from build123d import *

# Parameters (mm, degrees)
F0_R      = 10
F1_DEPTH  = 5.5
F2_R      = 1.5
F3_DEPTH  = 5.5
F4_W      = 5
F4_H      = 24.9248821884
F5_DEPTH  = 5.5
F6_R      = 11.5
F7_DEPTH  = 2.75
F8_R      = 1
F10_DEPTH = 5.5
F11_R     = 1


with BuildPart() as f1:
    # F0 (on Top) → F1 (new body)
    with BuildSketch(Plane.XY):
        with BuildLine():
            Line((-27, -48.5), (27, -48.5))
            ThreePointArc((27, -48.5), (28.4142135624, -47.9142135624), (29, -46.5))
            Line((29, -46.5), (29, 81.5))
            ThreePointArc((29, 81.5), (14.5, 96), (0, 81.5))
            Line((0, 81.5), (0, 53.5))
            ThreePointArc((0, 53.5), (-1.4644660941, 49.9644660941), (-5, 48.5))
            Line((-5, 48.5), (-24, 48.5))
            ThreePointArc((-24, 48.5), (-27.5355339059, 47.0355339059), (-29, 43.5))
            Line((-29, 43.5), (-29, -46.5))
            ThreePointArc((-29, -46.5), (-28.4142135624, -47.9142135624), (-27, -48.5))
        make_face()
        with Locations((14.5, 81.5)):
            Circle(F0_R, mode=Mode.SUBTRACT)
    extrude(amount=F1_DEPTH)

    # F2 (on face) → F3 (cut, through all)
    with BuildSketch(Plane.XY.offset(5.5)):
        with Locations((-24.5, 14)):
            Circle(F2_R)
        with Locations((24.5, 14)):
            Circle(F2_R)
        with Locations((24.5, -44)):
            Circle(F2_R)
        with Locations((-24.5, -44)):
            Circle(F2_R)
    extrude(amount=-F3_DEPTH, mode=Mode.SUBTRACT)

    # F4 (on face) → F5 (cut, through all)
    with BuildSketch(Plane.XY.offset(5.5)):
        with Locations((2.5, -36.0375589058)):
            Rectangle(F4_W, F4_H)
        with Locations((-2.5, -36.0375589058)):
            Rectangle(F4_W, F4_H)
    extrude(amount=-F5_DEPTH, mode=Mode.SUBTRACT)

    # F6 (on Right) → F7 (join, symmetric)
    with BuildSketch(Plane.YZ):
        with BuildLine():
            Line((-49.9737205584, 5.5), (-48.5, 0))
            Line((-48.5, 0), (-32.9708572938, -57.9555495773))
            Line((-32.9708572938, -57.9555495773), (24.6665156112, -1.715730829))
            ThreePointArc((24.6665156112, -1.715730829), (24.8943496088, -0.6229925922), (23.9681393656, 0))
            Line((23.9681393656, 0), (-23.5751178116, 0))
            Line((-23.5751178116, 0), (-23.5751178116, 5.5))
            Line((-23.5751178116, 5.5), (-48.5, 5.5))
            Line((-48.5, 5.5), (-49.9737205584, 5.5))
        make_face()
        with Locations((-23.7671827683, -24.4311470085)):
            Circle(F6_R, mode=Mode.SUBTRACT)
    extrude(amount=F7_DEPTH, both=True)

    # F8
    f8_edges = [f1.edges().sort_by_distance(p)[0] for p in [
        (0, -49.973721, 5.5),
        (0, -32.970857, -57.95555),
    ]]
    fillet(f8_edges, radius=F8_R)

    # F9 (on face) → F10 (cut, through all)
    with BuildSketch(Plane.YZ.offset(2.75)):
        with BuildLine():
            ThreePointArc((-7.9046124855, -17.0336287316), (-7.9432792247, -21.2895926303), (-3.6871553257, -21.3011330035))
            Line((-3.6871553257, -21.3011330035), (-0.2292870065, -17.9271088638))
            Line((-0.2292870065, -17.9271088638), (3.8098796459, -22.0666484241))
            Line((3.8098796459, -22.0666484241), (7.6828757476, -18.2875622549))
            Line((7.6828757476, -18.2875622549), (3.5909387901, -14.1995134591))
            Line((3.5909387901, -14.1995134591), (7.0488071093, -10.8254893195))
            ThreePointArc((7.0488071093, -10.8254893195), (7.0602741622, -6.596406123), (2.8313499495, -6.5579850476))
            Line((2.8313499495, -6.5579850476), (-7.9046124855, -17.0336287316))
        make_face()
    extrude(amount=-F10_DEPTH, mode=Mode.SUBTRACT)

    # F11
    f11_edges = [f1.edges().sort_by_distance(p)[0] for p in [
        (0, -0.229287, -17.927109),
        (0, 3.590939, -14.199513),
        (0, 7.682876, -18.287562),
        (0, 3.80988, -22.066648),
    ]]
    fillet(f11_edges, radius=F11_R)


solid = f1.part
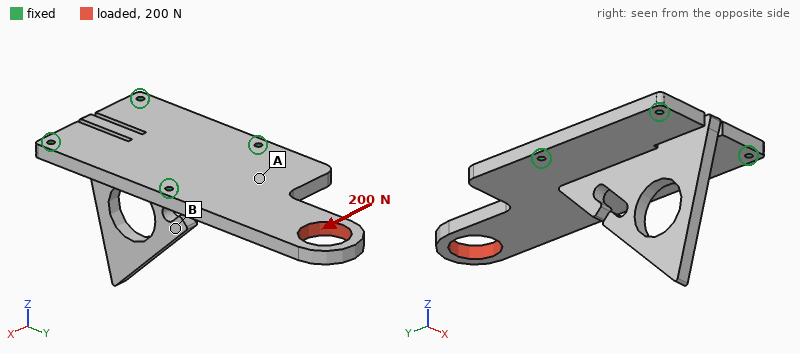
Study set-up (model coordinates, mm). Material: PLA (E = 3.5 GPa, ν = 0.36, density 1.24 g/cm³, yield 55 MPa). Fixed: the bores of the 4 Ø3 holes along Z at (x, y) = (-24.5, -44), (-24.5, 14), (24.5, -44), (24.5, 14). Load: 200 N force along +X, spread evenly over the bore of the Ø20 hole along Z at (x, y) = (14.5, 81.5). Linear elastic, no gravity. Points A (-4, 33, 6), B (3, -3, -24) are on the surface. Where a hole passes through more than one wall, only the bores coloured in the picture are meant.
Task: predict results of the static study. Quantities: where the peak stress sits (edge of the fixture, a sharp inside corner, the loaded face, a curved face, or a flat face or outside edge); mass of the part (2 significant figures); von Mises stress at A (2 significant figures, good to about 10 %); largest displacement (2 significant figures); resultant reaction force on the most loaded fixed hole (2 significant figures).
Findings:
a curved face
55 g
3.3 MPa
0.49 mm
280 N
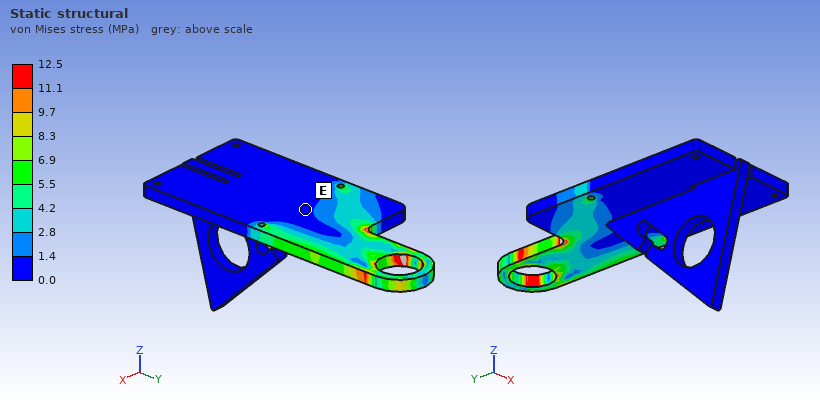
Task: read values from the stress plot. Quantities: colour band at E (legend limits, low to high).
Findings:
0.0 to 1.4 MPa
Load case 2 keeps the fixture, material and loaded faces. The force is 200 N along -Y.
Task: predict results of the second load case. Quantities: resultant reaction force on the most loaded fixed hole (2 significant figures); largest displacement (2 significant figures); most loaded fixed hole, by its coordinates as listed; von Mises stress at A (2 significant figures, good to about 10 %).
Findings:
140 N
65 µm
(24.5, 14)
0.37 MPa
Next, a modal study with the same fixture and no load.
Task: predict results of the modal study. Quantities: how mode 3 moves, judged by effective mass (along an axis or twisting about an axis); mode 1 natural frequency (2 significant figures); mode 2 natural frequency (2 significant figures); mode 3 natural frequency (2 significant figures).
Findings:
along Z
350 Hz
490 Hz
870 Hz
